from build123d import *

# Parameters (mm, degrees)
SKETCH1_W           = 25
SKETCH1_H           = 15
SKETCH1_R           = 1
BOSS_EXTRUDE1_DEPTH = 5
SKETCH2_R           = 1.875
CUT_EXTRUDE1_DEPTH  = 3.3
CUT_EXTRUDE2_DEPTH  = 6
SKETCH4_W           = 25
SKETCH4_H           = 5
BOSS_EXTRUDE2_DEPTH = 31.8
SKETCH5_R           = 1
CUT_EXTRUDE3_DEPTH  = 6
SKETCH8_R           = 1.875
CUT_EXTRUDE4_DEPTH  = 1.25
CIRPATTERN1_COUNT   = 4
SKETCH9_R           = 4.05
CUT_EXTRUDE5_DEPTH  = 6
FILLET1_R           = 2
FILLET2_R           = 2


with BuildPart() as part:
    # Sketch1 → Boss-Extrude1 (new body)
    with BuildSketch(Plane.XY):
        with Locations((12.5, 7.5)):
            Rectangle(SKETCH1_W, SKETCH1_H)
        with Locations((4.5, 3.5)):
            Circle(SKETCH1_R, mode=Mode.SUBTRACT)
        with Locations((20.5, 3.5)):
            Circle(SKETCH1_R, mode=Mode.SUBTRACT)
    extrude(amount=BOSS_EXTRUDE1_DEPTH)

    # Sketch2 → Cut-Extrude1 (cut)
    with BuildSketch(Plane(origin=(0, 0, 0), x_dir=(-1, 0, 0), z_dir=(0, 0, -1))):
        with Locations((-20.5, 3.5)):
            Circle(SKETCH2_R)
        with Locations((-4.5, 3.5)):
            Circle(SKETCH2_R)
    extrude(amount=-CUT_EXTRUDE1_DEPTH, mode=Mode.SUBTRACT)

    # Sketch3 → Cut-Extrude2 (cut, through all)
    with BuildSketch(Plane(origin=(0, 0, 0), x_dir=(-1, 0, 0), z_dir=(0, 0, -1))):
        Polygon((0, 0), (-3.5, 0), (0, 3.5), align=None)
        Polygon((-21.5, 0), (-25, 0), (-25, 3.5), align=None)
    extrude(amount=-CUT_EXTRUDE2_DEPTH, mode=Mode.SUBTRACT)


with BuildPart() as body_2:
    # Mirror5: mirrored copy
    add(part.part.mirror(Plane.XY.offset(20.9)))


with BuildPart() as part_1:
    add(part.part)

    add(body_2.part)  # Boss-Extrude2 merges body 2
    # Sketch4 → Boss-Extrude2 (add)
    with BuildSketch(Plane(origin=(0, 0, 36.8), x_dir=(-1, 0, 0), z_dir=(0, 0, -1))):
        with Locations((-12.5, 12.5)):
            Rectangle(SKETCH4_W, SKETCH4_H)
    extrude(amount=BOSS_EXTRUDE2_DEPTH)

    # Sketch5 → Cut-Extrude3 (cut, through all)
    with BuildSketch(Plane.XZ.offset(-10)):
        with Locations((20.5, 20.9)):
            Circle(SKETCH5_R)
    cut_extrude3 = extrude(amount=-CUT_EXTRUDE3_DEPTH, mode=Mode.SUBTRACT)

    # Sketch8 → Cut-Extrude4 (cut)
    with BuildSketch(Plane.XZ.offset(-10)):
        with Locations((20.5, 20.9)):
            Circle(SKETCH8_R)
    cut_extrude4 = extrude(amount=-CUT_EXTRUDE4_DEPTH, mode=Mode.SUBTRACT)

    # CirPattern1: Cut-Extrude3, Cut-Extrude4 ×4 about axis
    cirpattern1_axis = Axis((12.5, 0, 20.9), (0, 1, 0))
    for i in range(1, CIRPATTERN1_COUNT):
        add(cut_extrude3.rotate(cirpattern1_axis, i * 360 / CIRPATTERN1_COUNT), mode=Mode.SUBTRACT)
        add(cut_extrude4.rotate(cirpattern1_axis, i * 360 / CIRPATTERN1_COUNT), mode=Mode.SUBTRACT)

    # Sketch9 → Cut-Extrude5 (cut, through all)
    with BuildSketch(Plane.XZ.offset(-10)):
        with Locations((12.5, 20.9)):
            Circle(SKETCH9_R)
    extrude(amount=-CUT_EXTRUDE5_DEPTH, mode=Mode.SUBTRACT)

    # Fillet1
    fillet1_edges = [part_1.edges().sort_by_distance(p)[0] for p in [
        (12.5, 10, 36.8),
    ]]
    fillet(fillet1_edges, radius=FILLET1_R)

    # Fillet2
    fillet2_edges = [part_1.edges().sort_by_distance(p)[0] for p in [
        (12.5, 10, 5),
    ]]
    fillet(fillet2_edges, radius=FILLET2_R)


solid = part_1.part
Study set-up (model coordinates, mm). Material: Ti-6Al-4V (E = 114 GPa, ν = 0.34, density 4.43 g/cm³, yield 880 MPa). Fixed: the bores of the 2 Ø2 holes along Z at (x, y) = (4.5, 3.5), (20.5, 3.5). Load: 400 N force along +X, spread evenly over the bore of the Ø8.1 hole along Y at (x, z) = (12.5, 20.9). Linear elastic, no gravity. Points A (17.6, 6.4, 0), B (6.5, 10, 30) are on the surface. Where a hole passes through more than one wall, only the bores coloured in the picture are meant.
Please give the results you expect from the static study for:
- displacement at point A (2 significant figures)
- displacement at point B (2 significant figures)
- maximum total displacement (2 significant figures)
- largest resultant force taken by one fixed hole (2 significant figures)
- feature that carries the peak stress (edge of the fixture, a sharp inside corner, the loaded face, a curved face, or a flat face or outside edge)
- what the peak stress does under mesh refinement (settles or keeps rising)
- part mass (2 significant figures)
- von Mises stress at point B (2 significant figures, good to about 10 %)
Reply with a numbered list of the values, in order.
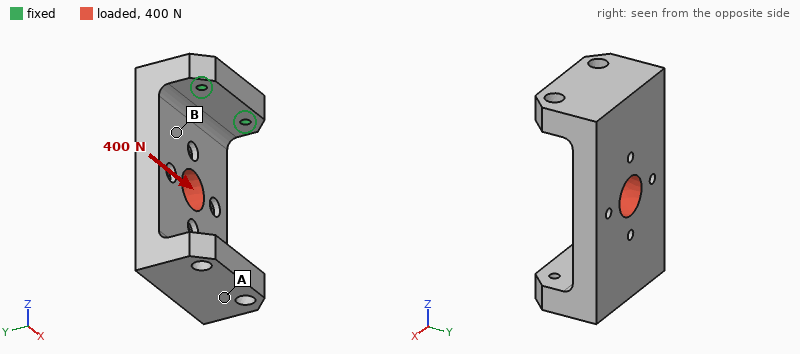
1. 47 µm
2. 13 µm
3. 50 µm
4. 490 N
5. edge of the fixture
6. keeps rising
7. 32 g
8. 17 MPa
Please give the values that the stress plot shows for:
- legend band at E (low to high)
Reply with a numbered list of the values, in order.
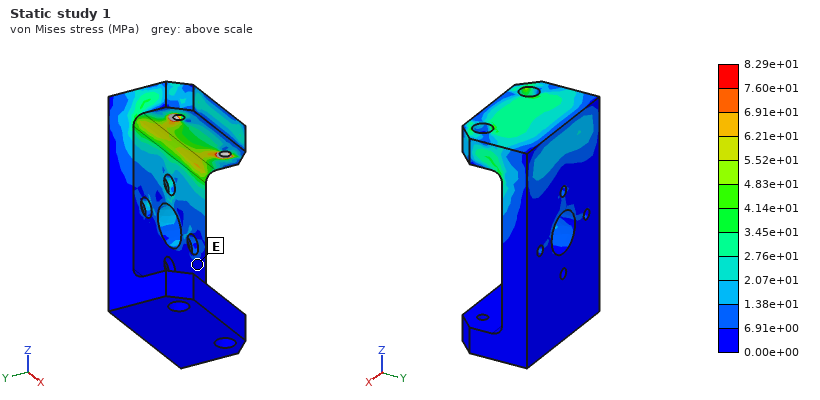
1. 0.00e+00 to 6.91e+00 MPa
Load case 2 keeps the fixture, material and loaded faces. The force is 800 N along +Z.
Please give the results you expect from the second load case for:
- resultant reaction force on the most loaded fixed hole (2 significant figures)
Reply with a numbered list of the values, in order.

1. 400 N
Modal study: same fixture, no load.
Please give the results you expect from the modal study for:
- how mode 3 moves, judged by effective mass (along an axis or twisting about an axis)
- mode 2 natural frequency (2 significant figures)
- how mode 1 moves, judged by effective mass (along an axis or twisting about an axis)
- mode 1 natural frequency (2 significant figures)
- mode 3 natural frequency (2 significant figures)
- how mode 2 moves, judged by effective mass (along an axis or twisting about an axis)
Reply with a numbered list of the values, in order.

1. along Z
2. 2800 Hz
3. along Y
4. 1000 Hz
5. 5100 Hz
6. along X
